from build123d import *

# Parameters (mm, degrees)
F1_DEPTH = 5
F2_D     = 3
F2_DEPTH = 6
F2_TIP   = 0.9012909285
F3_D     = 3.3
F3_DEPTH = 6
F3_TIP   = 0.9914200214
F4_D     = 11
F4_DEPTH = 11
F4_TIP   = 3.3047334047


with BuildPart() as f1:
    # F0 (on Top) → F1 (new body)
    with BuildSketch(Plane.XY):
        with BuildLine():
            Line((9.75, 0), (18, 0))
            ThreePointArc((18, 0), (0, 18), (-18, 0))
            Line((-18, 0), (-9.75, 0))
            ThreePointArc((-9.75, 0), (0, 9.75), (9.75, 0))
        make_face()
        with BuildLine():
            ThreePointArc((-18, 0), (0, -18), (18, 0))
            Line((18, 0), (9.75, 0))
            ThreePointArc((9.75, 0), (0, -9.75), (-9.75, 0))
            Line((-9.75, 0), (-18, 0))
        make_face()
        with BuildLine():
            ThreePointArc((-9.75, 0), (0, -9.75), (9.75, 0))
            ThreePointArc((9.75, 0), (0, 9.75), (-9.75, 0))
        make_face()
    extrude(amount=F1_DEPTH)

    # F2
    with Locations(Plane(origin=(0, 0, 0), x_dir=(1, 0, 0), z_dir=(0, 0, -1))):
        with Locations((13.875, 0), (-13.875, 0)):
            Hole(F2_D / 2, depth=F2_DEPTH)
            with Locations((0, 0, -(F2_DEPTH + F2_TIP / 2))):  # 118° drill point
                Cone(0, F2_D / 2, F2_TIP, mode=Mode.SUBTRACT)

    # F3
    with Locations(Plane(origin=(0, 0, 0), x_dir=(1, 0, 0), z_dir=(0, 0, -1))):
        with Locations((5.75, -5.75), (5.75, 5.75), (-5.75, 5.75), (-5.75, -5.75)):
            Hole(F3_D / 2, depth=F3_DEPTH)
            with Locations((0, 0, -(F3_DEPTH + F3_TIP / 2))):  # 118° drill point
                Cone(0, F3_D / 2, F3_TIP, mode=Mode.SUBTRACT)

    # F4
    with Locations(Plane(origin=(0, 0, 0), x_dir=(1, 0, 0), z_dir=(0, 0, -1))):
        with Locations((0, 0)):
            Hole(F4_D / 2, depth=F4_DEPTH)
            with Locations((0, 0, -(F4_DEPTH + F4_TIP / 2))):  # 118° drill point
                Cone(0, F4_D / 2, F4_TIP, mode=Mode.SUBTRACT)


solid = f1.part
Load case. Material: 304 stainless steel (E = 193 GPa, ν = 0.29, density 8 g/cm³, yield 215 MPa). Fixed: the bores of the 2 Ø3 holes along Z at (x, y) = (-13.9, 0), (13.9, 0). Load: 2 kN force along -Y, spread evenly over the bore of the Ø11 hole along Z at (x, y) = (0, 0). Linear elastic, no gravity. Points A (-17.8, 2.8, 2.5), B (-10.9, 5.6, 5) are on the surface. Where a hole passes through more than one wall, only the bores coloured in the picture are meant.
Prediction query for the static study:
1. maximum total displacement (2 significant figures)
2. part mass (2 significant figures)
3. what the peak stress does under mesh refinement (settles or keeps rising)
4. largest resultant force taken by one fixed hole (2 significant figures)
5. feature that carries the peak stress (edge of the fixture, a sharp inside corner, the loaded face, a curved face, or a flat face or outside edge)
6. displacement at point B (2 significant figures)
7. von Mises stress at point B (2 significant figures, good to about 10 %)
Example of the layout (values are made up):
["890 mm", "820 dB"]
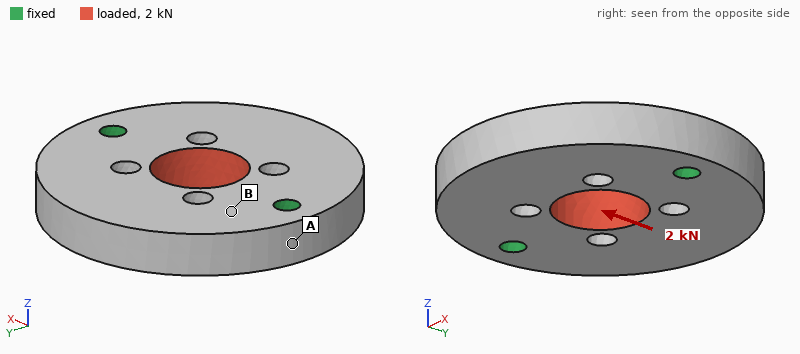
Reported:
["1.9 µm", "35 g", "keeps rising", "1.0 kN", "edge of the fixture", "0.68 µm", "18 MPa"]
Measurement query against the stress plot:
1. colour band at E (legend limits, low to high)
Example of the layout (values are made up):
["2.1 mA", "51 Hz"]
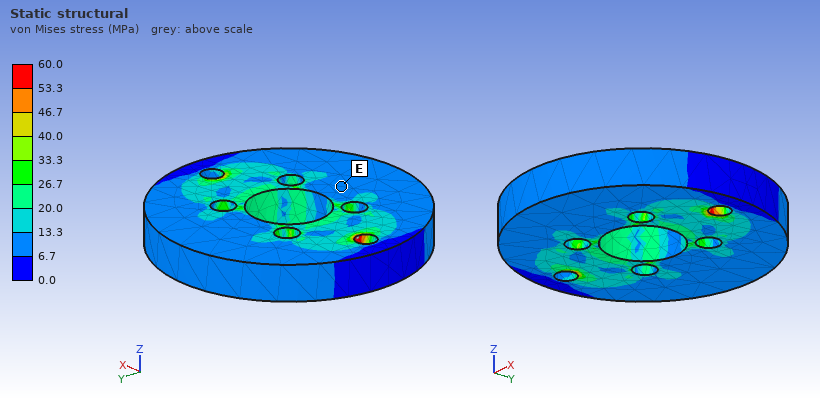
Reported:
["6.7 to 13.3 MPa"]
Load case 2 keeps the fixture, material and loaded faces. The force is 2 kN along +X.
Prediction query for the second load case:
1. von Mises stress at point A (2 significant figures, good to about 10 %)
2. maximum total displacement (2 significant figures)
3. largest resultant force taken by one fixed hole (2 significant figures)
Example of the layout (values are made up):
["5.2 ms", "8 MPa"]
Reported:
["10 MPa", "1.7 µm", "1.0 kN"]
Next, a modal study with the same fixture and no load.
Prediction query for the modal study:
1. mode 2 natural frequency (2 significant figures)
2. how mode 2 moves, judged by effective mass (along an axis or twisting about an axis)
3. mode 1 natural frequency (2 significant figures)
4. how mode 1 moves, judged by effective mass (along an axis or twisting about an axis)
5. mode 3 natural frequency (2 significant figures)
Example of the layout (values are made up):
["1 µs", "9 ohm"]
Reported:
["12 kHz", "along Z", "10 kHz", "twisting about X", "26 kHz"]
